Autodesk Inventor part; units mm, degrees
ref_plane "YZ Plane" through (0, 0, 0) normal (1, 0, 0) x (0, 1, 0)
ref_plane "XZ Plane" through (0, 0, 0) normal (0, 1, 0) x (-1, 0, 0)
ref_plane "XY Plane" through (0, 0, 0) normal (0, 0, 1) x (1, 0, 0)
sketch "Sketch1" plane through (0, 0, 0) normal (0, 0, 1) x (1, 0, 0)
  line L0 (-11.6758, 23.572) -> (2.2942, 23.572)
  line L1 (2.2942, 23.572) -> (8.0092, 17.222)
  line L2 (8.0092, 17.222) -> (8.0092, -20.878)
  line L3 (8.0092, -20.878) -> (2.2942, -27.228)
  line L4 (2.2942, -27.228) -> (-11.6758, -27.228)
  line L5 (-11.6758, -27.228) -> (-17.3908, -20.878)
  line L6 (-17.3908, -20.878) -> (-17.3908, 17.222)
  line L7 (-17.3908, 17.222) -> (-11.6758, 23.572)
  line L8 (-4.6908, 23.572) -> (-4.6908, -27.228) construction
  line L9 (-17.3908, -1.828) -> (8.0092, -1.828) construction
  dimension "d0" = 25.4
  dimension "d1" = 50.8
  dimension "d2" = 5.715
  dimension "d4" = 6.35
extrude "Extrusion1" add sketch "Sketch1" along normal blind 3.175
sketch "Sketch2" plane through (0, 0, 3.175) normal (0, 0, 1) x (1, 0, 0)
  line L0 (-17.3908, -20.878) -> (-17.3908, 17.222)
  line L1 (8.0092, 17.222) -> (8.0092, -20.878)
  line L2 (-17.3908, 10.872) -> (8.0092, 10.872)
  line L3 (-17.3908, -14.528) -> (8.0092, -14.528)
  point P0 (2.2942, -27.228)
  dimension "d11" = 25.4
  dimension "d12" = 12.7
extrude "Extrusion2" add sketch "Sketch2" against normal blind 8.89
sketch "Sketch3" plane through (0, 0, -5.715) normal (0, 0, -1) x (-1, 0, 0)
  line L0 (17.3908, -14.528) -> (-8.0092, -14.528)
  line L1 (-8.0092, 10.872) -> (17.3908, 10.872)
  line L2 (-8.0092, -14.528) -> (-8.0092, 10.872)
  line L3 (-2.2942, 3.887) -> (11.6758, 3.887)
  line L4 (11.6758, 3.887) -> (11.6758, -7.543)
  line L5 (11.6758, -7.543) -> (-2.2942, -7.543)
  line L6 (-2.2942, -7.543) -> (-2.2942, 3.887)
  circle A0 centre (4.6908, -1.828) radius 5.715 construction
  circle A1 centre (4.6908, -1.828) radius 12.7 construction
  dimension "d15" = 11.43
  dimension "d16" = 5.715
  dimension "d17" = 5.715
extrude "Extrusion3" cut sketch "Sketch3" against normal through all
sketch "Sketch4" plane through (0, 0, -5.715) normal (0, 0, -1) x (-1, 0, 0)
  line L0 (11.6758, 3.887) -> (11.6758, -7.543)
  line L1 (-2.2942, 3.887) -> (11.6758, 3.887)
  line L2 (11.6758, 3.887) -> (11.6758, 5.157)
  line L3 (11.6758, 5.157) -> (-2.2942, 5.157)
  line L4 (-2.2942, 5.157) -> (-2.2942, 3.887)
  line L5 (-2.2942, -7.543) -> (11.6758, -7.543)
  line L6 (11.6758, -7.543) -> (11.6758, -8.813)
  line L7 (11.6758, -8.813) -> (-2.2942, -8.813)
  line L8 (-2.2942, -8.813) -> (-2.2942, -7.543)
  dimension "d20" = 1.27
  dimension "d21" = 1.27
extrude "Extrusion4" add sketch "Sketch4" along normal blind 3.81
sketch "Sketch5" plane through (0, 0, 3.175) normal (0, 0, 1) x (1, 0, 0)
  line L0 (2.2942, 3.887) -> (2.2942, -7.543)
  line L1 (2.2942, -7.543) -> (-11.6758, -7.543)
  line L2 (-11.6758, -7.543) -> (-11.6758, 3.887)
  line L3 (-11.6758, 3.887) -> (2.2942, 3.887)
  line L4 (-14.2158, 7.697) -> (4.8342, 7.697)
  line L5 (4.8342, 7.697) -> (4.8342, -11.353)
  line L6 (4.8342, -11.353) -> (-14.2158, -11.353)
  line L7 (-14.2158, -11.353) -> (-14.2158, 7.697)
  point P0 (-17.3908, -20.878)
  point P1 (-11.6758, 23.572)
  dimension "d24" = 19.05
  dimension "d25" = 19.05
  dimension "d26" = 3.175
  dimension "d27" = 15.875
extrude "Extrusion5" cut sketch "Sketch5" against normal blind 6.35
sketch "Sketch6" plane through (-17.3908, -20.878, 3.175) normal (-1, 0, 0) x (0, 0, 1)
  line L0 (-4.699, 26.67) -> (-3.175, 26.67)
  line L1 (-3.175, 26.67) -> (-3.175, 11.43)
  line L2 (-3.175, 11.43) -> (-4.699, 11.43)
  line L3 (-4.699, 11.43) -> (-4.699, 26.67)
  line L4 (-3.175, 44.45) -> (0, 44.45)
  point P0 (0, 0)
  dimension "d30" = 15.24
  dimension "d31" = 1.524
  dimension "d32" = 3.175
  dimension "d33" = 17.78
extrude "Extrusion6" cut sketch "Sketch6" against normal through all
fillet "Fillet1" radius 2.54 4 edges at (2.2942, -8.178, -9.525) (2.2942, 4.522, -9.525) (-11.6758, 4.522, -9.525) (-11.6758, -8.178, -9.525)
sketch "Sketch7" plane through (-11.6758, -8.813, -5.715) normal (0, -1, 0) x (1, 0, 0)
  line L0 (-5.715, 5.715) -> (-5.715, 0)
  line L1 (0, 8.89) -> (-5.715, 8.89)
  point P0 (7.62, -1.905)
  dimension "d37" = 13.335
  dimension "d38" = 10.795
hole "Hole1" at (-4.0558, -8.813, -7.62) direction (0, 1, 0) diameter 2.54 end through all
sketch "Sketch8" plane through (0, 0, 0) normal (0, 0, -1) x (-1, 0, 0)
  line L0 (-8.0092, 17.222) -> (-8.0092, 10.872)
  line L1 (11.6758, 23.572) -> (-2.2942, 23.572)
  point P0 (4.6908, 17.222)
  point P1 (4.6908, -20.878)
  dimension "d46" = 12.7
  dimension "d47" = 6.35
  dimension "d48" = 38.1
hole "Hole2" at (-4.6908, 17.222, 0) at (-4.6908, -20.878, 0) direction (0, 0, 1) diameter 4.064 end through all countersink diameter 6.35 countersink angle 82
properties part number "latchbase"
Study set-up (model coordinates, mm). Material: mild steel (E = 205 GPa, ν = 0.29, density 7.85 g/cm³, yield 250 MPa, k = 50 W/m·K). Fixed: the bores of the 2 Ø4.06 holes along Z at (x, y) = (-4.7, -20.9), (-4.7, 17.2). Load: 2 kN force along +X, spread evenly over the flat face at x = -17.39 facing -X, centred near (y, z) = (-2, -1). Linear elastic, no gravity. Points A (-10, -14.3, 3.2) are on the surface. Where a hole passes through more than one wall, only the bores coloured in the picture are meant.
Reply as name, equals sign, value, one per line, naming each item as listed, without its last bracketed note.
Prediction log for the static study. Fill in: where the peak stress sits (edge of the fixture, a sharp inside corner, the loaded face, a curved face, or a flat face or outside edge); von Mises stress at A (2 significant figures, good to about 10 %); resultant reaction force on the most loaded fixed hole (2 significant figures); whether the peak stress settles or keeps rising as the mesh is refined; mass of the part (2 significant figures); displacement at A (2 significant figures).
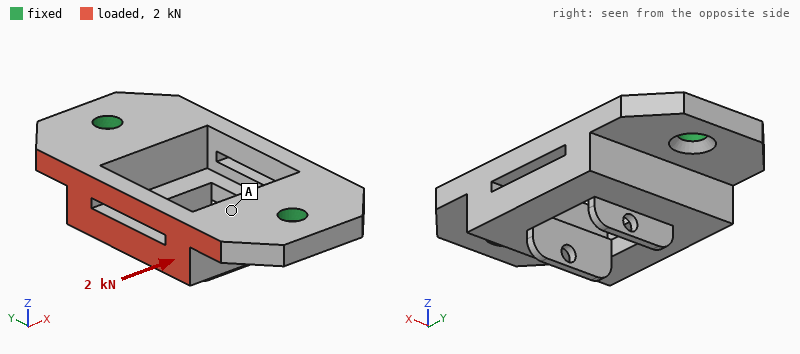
where the peak stress sits = edge of the fixture
von Mises stress at A = 23 MPa
resultant reaction force on the most loaded fixed hole = 1.0 kN
whether the peak stress settles or keeps rising as the mesh is refined = keeps rising
mass of the part = 37 g
displacement at A = 7.2 µm
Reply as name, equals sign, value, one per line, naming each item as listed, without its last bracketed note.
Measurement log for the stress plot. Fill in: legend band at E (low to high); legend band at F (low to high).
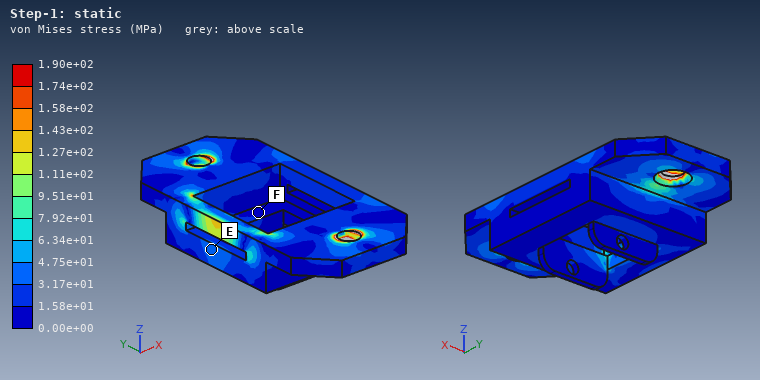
legend band at E = 3.17e+01 to 4.75e+01 MPa
legend band at F = 0.00e+00 to 1.58e+01 MPa
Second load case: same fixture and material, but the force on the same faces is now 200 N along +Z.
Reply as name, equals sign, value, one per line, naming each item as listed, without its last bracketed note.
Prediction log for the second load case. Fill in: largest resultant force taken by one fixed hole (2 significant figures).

largest resultant force taken by one fixed hole = 140 N
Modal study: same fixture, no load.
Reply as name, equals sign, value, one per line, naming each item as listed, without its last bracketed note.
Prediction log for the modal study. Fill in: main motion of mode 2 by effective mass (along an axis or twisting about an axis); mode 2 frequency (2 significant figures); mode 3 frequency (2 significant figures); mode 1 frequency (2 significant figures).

main motion of mode 2 by effective mass = along Z
mode 2 frequency = 13 kHz
mode 3 frequency = 14 kHz
mode 1 frequency = 6300 Hz
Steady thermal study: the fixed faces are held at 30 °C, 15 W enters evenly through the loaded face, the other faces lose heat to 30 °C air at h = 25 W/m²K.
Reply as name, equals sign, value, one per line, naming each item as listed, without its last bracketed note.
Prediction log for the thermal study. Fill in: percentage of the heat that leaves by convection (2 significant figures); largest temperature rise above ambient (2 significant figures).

percentage of the heat that leaves by convection = 11 %
largest temperature rise above ambient = 55 K
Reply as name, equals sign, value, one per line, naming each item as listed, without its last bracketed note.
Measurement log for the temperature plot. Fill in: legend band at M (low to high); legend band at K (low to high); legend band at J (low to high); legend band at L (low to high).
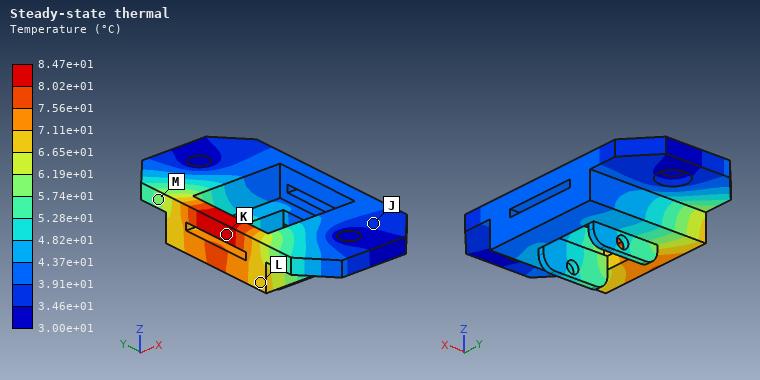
legend band at M = 5.74e+01 to 6.19e+01 °C
legend band at K = 8.02e+01 to 8.47e+01 °C
legend band at J = 3.46e+01 to 3.91e+01 °C
legend band at L = 6.65e+01 to 7.11e+01 °C
